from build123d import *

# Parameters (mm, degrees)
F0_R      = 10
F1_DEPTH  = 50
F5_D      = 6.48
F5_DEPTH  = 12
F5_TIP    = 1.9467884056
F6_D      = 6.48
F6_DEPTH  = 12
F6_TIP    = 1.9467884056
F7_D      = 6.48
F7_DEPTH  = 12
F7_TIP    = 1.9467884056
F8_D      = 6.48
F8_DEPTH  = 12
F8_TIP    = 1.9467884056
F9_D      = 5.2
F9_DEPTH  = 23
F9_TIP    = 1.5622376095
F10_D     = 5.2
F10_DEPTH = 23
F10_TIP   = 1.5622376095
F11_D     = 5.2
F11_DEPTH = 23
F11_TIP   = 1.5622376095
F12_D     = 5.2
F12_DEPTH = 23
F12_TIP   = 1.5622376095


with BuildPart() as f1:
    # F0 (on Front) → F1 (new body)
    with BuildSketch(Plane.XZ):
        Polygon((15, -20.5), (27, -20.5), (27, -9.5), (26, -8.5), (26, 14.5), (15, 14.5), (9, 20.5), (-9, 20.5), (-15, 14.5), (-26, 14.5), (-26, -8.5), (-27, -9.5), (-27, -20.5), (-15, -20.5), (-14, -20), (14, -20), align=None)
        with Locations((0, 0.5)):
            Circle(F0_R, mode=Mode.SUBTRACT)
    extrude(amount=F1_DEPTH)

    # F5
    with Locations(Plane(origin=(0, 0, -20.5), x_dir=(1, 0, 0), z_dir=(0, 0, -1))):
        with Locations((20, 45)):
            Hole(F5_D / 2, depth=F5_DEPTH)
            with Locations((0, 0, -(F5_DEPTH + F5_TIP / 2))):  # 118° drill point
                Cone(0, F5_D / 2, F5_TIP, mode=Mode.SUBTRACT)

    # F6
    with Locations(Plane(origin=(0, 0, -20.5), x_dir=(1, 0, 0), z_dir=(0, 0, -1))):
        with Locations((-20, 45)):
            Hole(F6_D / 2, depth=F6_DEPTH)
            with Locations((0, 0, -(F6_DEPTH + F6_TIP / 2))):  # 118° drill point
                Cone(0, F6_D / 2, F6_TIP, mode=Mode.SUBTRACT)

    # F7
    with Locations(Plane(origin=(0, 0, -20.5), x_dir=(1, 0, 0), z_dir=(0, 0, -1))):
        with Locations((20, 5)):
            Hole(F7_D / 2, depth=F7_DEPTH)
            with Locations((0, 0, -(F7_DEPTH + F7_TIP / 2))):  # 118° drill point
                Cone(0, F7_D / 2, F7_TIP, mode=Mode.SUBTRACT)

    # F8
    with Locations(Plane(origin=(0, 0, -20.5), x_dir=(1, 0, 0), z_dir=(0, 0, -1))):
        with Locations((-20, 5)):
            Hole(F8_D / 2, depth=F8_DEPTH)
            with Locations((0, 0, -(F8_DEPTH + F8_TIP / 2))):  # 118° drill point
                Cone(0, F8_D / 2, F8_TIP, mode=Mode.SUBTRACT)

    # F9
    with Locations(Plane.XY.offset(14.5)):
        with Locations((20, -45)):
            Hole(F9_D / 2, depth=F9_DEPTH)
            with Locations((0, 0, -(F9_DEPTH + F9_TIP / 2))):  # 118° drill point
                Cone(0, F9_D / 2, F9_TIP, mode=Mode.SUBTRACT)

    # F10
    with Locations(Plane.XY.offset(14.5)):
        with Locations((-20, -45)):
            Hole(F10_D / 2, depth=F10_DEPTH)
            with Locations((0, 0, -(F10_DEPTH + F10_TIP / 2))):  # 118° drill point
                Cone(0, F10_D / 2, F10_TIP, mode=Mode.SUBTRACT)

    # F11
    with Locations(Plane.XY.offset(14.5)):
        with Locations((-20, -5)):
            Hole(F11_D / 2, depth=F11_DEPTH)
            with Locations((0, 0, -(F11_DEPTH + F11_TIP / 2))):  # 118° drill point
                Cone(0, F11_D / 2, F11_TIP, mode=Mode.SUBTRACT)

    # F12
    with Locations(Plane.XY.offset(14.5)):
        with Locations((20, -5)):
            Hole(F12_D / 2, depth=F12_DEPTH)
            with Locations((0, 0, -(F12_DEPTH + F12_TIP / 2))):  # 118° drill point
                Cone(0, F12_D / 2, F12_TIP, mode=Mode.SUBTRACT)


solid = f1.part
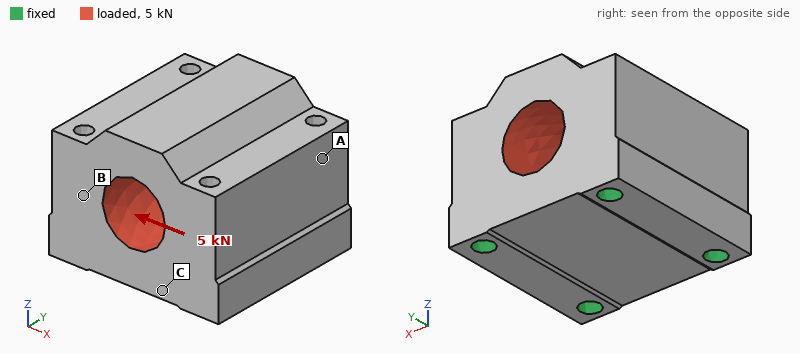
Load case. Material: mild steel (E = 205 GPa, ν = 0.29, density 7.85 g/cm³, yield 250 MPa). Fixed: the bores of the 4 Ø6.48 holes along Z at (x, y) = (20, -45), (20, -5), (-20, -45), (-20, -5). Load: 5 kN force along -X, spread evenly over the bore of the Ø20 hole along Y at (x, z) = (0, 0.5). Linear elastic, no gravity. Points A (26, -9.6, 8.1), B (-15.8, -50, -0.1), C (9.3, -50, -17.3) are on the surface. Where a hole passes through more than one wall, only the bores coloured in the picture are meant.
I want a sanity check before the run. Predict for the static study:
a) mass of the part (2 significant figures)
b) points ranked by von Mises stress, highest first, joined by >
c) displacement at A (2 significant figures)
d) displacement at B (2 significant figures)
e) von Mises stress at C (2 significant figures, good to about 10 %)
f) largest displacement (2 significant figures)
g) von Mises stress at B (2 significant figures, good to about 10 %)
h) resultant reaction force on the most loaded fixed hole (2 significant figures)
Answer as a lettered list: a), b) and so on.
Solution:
a) 620 g
b) B > C > A
c) 1.4 µm
d) 0.77 µm
e) 3.3 MPa
f) 1.7 µm
g) 7.3 MPa
h) 1.5 kN
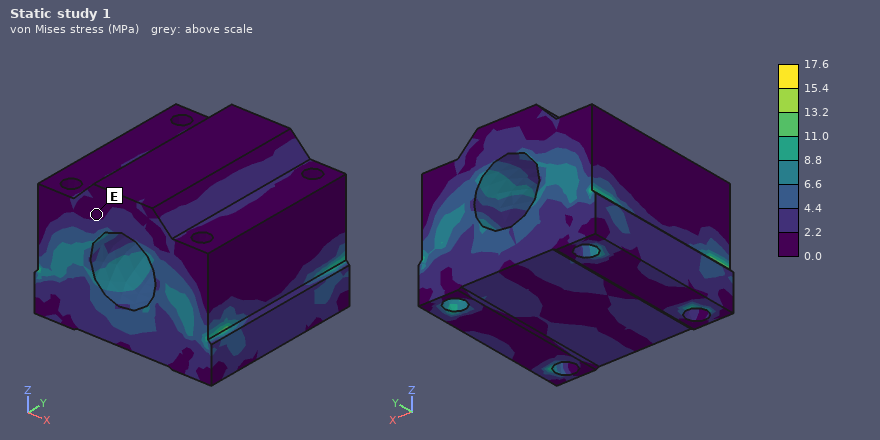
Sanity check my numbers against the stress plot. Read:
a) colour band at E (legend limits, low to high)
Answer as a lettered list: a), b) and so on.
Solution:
a) 0.0 to 2.2 MPa
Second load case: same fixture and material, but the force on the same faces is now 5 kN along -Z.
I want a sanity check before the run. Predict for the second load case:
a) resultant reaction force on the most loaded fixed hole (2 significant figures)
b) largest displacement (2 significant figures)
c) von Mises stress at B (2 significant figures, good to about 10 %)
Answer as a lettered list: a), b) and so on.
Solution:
a) 1.3 kN
b) 0.72 µm
c) 5.2 MPa
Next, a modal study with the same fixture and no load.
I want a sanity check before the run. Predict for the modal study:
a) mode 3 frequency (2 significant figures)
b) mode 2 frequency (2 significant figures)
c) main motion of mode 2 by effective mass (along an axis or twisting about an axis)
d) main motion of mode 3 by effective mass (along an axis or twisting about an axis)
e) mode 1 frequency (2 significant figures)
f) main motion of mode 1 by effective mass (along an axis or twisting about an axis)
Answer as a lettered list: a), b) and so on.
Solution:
a) 21 kHz
b) 17 kHz
c) along Y
d) twisting about Z
e) 13 kHz
f) along X
